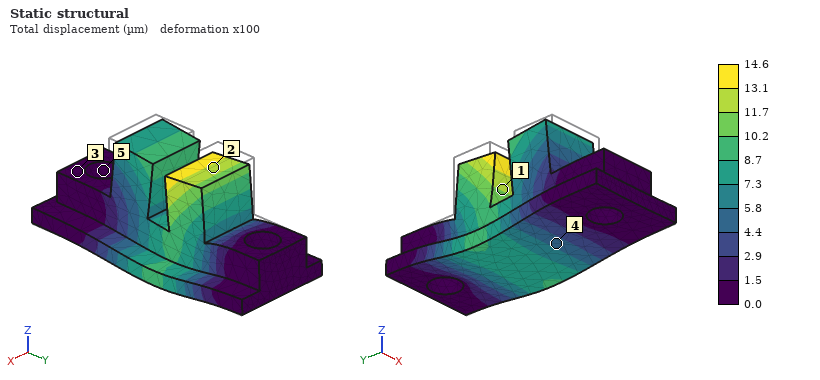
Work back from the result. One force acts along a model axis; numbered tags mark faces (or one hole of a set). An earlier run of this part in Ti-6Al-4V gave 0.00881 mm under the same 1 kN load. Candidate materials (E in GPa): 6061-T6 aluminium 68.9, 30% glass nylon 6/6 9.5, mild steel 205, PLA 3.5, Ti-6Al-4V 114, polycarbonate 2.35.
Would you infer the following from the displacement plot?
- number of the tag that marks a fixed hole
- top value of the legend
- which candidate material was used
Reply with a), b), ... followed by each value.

a) 5
b) 14.6 µm
c) 6061-T6 aluminium
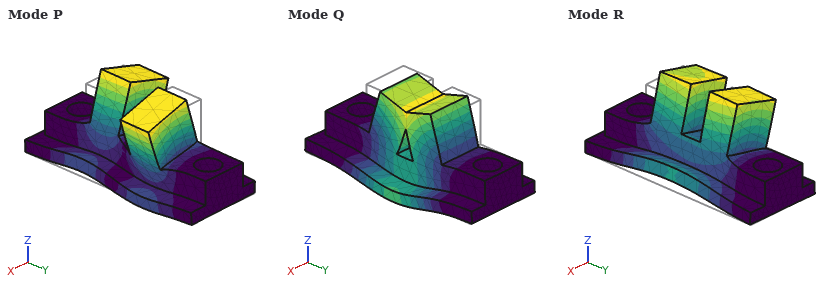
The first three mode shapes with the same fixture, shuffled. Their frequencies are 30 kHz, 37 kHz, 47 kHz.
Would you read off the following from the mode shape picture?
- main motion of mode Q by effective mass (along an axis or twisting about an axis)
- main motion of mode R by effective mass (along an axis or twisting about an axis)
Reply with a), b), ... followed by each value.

a) along Z
b) along X
